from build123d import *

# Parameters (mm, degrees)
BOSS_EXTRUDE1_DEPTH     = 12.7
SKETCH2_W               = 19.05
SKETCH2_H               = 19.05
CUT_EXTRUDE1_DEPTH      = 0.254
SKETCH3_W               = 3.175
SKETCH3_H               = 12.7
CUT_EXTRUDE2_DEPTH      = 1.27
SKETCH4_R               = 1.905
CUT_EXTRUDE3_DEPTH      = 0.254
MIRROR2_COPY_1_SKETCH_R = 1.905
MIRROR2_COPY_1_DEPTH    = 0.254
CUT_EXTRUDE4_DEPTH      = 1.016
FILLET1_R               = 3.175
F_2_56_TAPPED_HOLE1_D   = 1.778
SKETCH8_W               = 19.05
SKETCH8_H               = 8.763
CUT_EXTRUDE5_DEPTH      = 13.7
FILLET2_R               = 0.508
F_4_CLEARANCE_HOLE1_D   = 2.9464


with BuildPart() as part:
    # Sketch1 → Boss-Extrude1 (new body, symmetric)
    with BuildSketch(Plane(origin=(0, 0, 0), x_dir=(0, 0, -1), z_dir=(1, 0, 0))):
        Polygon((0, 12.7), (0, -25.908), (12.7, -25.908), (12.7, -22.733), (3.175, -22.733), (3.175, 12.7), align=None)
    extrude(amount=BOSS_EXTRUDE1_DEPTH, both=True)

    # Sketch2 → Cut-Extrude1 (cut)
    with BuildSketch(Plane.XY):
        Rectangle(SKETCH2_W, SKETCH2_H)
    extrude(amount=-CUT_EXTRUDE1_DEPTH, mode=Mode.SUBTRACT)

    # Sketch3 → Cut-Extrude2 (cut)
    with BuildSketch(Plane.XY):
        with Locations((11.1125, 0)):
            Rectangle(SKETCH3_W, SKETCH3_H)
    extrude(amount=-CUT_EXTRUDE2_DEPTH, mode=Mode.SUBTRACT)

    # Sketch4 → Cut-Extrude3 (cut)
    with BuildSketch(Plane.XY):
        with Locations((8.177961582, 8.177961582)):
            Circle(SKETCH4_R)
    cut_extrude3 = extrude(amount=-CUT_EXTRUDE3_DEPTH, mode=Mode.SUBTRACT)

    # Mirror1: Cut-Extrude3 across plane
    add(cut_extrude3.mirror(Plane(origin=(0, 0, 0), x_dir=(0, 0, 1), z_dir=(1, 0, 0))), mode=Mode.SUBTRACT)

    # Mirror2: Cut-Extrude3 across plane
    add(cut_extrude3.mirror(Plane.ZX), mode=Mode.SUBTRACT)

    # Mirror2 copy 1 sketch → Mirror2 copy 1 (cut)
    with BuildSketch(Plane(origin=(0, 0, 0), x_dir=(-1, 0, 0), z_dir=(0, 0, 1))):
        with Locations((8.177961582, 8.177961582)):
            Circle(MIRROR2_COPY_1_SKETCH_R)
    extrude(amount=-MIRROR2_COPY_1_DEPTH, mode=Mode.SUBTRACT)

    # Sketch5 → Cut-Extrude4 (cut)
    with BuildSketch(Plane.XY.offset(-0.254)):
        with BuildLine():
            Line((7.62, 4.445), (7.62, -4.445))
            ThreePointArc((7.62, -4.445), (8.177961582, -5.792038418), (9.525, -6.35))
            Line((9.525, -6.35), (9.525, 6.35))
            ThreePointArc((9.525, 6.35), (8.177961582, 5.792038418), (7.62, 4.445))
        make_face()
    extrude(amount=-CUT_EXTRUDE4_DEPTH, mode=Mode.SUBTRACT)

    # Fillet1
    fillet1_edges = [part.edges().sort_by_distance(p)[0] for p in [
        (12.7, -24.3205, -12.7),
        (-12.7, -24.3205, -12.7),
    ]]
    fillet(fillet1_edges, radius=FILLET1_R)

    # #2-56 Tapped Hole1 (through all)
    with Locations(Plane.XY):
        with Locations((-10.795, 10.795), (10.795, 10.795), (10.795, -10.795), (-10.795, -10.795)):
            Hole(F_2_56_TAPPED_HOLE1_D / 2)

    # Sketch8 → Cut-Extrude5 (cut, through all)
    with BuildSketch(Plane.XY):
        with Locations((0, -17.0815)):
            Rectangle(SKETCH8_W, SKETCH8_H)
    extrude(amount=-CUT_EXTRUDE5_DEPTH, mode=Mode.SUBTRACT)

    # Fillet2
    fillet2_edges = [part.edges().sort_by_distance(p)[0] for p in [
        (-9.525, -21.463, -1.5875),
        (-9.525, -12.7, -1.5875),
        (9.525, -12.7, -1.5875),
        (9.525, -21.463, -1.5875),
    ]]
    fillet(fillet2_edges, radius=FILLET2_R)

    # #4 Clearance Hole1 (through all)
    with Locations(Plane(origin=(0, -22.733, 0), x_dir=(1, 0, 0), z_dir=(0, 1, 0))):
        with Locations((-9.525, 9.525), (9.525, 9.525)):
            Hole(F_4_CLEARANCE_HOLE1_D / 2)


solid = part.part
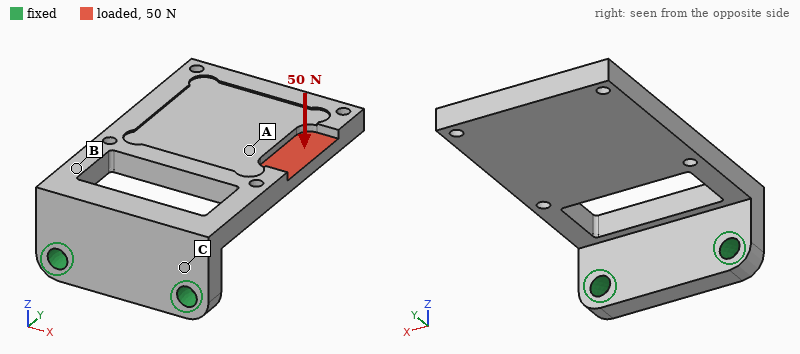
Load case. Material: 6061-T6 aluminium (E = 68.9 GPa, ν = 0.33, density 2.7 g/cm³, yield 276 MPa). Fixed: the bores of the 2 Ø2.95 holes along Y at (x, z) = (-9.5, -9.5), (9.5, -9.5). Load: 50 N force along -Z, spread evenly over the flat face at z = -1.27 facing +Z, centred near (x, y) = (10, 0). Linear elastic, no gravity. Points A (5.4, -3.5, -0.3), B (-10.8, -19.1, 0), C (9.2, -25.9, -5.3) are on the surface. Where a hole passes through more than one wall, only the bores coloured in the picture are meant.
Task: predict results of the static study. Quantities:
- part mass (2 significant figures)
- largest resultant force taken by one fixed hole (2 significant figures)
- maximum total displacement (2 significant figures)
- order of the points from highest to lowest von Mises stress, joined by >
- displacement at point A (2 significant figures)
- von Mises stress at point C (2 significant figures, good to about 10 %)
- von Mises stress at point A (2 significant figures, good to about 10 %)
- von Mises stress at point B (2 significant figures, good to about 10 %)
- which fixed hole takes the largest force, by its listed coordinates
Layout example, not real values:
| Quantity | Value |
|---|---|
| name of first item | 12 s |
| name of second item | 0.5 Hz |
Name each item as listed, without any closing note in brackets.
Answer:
| Quantity | Value |
|---|---|
| part mass | 8.4 g |
| largest resultant force taken by one fixed hole | 51 N |
| maximum total displacement | 0.45 mm |
| order of the points from highest to lowest von Mises stress, joined by > | B > C > A |
| displacement at point A | 0.21 mm |
| von Mises stress at point C | 43 MPa |
| von Mises stress at point A | 16 MPa |
| von Mises stress at point B | 78 MPa |
| which fixed hole takes the largest force, by its listed coordinates | (9.5, -9.5) |
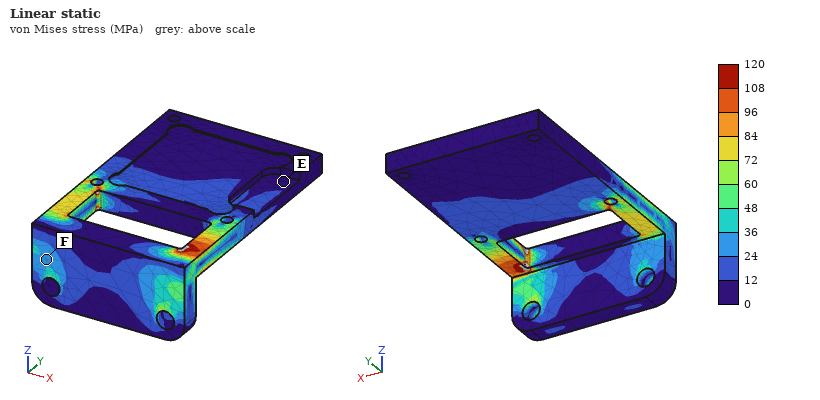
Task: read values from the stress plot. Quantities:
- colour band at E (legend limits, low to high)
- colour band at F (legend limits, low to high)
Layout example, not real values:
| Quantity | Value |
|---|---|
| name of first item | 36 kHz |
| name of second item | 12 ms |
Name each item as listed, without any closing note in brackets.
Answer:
| Quantity | Value |
|---|---|
| colour band at E | 0 to 12 MPa |
| colour band at F | 24 to 36 MPa |
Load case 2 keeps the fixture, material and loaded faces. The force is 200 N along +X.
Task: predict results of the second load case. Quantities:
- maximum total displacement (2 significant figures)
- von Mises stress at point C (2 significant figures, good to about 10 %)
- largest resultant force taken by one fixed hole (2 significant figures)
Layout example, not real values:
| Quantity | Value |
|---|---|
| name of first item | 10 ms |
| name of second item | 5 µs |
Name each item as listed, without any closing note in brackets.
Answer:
| Quantity | Value |
|---|---|
| maximum total displacement | 0.10 mm |
| von Mises stress at point C | 48 MPa |
| largest resultant force taken by one fixed hole | 260 N |
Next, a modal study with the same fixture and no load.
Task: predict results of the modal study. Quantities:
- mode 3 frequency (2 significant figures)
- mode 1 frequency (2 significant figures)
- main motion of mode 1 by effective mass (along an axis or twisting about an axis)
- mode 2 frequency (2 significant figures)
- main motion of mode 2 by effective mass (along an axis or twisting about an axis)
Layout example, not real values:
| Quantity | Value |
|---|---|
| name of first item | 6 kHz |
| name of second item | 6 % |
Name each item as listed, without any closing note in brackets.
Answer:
| Quantity | Value |
|---|---|
| mode 3 frequency | 4600 Hz |
| mode 1 frequency | 930 Hz |
| main motion of mode 1 by effective mass | along Z |
| mode 2 frequency | 3400 Hz |
| main motion of mode 2 by effective mass | along X |
